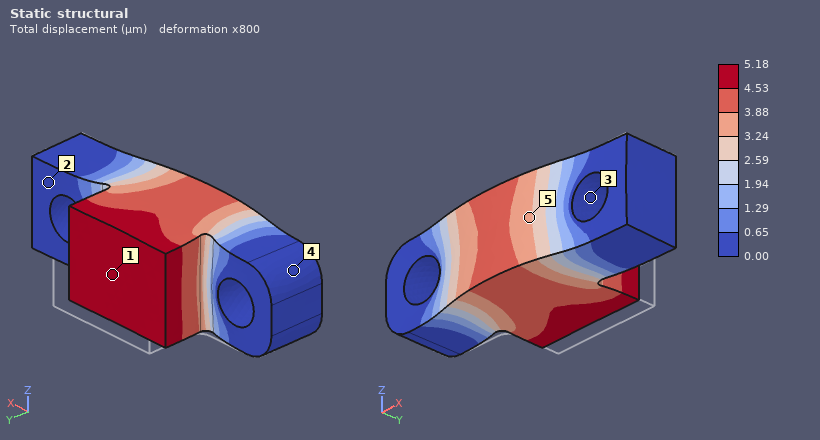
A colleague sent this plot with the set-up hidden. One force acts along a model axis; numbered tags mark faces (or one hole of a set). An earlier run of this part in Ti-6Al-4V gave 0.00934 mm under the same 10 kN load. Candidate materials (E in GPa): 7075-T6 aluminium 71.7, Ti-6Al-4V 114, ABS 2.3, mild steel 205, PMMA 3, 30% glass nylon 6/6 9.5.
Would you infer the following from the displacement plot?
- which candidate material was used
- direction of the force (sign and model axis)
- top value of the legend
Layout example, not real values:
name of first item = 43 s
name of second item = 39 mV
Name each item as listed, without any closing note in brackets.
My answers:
which candidate material was used = mild steel
direction of the force = -Y
top value of the legend = 5.18 µm
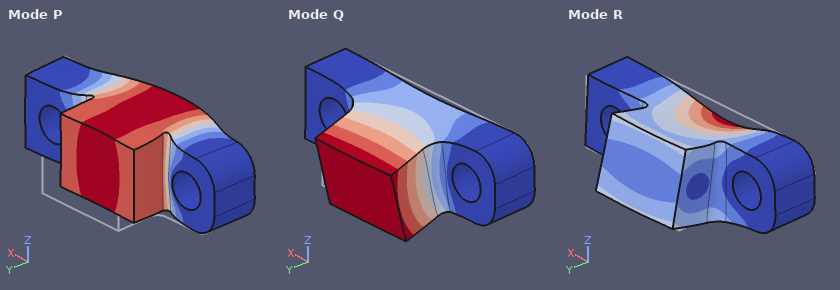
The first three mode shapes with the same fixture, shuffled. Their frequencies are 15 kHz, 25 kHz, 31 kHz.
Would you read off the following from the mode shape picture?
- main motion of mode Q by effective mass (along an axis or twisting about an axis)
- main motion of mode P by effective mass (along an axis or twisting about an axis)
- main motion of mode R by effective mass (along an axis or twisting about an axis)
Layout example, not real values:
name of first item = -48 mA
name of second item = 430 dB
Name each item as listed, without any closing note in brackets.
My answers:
main motion of mode Q by effective mass = along Z
main motion of mode P by effective mass = along Y
main motion of mode R by effective mass = along Z
